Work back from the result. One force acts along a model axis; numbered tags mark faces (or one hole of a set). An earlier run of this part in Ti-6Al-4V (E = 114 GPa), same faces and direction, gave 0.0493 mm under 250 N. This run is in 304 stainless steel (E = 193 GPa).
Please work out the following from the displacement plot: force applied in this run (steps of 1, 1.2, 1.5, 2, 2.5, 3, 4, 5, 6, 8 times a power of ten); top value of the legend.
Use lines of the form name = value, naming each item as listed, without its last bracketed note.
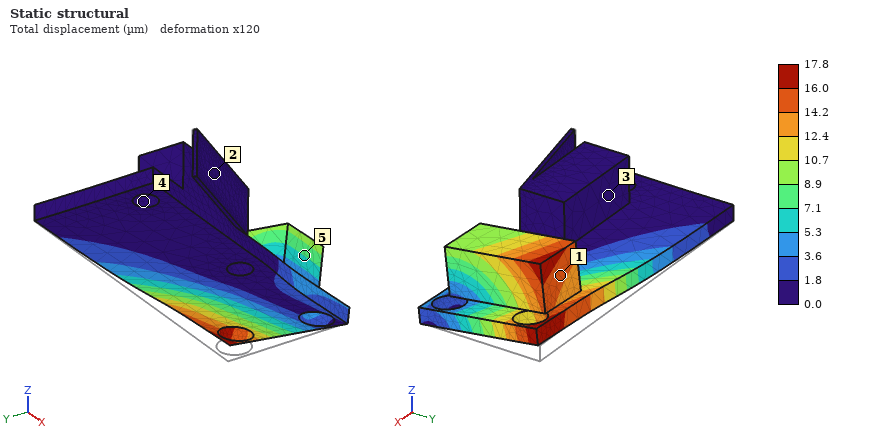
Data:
force applied in this run = 150 N
top value of the legend = 17.8 µm
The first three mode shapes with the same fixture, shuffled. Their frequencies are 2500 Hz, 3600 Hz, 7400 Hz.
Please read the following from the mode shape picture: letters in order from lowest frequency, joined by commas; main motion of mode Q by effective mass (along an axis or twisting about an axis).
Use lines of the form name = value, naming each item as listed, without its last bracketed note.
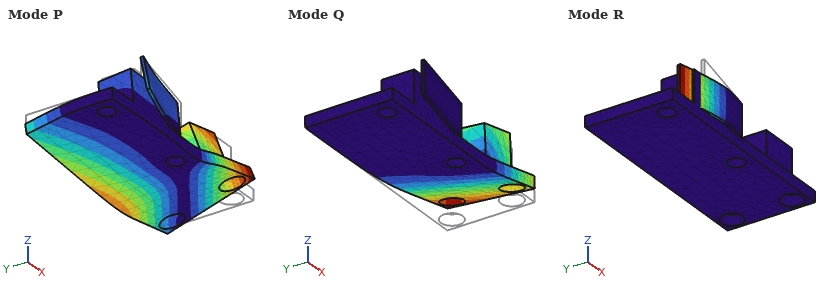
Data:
letters in order from lowest frequency, joined by commas = R, Q, P
main motion of mode Q by effective mass = along Z
